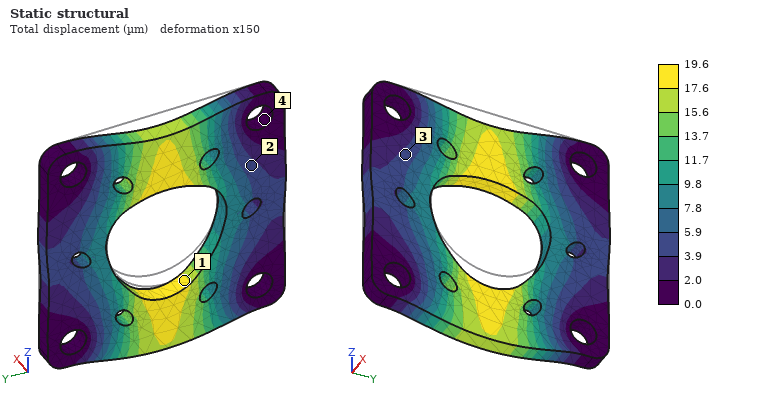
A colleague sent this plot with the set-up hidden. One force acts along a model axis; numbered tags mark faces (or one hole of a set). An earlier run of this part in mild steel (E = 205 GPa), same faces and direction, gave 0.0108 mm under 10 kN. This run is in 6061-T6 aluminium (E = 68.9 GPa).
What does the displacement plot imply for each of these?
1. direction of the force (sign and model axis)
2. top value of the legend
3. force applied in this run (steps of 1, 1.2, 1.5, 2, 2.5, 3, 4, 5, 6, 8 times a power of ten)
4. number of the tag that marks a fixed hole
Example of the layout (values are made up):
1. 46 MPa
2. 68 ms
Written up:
1. -Z
2. 19.6 µm
3. 6 kN
4. 4
